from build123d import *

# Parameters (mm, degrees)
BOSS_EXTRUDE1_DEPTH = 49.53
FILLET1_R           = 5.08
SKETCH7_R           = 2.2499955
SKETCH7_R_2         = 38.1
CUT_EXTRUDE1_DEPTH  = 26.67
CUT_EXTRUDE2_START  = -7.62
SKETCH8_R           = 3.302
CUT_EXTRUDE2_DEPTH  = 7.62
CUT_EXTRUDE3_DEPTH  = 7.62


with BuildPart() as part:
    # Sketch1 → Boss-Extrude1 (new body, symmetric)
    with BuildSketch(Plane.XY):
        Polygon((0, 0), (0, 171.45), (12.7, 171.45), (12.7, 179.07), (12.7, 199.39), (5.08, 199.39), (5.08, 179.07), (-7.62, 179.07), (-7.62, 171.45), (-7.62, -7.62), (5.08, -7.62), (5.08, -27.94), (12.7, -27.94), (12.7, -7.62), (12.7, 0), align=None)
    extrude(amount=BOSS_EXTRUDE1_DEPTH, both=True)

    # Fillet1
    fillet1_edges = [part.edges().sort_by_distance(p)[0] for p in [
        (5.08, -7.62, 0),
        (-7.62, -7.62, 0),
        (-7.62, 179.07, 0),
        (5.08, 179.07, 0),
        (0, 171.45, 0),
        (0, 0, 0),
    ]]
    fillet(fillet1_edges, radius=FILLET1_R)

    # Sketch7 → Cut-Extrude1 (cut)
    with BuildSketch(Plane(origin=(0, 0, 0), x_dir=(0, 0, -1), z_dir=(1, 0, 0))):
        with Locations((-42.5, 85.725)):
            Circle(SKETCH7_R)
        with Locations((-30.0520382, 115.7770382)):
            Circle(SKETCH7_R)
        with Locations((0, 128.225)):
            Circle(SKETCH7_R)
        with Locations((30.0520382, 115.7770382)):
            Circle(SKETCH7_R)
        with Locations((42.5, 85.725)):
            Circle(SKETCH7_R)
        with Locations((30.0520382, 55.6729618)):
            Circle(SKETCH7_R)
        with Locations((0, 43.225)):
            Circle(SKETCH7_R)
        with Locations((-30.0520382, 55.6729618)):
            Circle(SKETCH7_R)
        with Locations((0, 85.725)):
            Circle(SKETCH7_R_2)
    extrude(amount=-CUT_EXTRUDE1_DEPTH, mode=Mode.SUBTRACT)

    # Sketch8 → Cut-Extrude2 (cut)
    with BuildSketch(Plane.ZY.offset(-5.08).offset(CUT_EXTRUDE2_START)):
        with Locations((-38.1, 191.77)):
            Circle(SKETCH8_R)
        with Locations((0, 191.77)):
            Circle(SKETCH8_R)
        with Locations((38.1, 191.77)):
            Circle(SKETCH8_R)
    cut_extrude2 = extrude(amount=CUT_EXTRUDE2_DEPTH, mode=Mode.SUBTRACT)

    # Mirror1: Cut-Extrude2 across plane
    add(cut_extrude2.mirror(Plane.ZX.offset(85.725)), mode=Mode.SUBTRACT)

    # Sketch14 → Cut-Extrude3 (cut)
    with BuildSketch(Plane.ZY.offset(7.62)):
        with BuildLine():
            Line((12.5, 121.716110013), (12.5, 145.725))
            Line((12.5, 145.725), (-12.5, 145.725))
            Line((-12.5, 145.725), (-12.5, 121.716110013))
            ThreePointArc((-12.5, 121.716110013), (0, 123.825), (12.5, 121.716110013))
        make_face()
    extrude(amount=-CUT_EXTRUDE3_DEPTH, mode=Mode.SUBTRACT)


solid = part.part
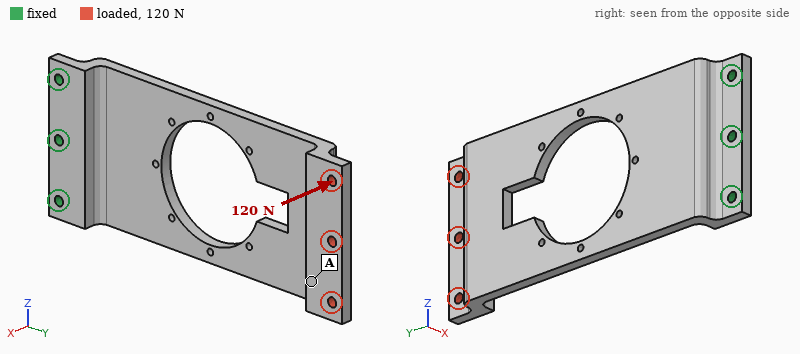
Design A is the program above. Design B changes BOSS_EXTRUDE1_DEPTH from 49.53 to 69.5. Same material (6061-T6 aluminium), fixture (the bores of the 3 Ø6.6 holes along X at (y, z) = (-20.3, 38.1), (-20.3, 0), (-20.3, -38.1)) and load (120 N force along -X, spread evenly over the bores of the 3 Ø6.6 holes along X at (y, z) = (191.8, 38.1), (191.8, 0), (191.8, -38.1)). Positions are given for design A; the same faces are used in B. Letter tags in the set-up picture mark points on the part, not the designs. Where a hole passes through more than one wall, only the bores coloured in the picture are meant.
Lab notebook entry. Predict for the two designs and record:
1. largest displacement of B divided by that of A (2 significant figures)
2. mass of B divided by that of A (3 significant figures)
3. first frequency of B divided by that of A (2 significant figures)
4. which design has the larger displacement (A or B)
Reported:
0.55
1.51
1.1
A
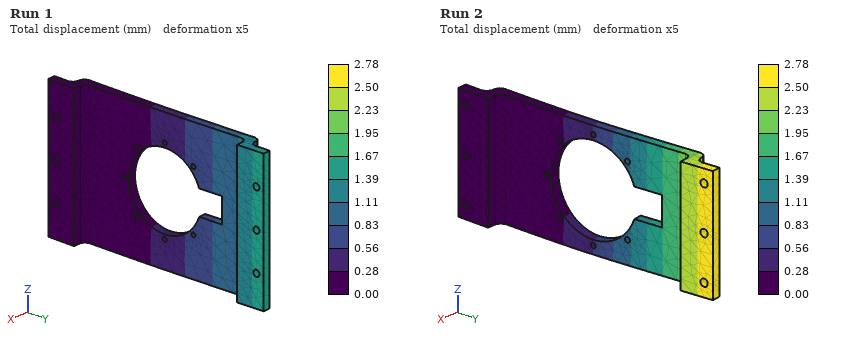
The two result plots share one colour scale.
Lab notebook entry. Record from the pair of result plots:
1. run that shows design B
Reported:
Run 1
